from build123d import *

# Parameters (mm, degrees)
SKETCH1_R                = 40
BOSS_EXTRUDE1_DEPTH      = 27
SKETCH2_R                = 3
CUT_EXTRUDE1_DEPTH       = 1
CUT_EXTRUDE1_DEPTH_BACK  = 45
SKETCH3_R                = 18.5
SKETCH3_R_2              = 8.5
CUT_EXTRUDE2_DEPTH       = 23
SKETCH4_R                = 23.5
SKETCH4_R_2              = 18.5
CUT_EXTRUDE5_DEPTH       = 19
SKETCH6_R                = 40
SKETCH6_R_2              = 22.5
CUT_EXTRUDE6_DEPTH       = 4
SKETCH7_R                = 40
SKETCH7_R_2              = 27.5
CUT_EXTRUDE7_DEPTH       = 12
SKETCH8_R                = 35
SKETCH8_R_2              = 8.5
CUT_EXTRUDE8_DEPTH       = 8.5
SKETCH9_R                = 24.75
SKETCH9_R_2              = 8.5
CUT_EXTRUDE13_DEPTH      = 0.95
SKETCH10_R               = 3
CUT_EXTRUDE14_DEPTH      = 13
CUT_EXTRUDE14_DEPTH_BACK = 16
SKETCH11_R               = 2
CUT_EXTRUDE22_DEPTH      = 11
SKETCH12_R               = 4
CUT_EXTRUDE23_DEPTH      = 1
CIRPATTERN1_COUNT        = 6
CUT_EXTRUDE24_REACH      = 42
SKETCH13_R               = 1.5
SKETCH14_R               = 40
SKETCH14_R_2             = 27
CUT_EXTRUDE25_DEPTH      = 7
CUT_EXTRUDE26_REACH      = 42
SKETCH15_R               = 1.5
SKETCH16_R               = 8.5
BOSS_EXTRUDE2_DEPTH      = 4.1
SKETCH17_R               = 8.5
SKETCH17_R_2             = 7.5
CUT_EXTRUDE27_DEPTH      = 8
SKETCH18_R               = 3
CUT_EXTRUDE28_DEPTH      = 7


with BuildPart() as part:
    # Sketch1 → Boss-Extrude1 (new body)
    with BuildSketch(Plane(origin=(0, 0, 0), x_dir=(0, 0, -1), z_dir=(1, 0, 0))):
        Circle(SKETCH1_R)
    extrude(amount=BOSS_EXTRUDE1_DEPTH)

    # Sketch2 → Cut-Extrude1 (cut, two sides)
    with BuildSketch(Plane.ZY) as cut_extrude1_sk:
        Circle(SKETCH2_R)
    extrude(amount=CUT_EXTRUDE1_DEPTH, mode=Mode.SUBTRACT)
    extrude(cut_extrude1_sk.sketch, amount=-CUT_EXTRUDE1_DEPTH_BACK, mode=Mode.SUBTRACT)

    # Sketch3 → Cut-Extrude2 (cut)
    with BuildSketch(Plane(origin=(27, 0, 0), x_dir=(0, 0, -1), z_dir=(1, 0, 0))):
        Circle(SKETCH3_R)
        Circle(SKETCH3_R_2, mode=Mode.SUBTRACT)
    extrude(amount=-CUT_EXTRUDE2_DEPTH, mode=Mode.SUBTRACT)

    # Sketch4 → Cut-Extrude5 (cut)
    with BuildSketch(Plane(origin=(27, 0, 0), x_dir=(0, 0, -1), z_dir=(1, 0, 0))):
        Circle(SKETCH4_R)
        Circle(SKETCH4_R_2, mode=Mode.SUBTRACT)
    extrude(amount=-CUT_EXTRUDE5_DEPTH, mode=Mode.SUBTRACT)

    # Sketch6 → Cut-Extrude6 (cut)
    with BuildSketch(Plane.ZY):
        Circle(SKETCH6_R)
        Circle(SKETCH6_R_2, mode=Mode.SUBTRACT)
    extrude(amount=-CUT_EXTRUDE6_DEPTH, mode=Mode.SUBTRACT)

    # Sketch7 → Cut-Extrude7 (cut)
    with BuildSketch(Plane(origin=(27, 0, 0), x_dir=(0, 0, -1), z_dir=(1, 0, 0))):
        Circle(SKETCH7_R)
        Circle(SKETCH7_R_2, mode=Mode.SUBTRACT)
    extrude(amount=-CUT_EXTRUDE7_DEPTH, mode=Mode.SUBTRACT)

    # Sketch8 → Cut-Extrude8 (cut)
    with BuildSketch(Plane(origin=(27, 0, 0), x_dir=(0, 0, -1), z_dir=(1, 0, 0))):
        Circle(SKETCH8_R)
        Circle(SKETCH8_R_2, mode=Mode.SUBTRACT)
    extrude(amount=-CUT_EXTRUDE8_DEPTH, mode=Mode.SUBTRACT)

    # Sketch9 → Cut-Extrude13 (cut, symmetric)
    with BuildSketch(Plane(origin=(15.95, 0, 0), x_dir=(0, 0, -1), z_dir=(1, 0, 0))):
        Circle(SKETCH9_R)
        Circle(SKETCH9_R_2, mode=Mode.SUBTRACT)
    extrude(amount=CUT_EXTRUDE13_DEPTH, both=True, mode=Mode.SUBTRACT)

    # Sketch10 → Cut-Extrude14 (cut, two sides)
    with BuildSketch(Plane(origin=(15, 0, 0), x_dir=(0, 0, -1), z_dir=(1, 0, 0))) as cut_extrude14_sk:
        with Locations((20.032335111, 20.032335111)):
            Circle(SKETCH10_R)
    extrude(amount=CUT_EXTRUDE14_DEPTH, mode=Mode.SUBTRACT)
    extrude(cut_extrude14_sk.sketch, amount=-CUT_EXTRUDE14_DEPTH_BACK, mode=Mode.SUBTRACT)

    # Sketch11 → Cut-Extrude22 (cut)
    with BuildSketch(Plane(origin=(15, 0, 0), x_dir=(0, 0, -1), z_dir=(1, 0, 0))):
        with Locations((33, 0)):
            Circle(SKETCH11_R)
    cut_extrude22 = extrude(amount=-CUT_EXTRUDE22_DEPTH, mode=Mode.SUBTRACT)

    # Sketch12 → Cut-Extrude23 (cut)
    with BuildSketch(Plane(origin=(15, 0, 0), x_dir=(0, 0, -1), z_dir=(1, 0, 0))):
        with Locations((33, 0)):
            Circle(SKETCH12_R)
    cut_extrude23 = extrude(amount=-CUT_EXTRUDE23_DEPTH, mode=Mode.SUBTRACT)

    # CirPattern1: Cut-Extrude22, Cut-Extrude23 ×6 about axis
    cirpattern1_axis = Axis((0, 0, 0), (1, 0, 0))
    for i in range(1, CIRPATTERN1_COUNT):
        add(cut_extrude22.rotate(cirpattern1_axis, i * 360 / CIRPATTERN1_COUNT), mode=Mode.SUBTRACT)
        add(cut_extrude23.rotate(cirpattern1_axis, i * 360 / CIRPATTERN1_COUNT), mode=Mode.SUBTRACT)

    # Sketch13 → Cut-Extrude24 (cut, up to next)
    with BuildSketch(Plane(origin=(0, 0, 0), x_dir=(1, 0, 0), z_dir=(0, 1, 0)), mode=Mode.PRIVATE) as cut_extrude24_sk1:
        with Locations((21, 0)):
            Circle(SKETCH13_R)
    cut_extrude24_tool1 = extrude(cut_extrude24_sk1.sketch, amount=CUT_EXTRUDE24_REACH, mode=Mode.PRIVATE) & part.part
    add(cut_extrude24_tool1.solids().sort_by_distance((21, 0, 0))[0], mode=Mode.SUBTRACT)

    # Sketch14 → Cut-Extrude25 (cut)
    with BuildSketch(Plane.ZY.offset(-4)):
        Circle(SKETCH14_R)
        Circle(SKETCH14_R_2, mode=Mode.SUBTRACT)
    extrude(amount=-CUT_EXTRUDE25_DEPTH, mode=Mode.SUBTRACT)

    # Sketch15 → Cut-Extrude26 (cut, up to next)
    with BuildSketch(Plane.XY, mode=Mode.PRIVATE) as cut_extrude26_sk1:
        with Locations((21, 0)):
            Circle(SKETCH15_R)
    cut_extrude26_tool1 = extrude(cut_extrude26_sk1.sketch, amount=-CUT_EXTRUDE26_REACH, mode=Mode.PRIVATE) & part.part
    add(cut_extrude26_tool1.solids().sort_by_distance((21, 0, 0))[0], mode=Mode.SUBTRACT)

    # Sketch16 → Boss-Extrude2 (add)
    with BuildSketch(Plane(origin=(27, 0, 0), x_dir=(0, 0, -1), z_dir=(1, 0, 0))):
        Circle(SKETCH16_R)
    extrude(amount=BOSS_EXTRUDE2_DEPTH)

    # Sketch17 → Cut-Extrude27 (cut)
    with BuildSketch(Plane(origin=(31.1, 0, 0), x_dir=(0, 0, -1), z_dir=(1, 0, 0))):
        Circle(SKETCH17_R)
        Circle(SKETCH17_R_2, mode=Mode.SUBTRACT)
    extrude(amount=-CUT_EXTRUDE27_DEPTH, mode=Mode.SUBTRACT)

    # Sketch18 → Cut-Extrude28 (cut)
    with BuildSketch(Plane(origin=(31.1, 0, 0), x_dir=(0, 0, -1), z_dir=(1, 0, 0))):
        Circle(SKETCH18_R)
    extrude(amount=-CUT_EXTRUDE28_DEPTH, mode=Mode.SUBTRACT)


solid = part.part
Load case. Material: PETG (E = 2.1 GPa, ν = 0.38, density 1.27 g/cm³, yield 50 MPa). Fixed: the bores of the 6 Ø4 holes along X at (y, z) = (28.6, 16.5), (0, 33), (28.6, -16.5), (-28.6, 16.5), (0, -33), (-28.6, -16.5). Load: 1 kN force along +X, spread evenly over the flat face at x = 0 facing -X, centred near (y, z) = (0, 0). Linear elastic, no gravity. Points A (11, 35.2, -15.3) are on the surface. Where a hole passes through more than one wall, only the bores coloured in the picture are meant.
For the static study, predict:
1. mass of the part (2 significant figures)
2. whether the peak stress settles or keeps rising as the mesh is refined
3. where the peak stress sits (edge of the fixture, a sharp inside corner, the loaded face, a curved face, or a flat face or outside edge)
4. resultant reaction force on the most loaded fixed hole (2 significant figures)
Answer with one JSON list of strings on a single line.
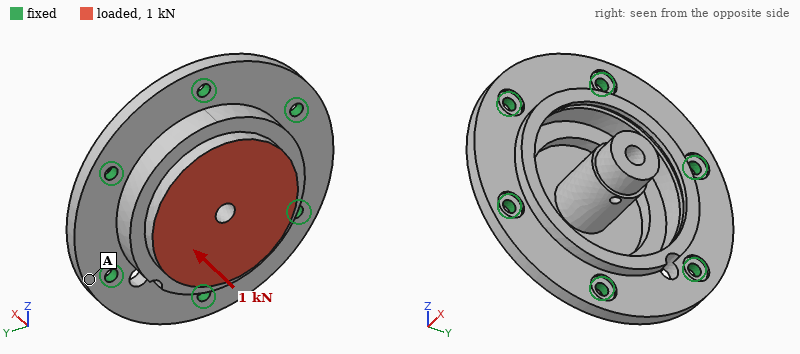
["41 g", "keeps rising", "edge of the fixture", "210 N"]
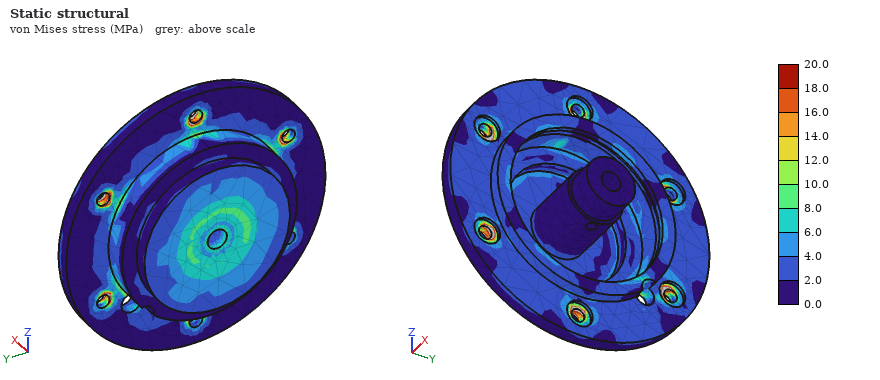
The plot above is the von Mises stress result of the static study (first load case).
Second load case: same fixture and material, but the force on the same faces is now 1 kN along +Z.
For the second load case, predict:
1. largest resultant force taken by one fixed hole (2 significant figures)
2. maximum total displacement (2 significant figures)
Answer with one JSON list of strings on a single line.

["220 N", "0.16 mm"]
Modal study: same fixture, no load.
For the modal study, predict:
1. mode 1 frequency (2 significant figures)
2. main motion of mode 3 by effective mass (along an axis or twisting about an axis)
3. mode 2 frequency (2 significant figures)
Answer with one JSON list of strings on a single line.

["1700 Hz", "along X", "1700 Hz"]
